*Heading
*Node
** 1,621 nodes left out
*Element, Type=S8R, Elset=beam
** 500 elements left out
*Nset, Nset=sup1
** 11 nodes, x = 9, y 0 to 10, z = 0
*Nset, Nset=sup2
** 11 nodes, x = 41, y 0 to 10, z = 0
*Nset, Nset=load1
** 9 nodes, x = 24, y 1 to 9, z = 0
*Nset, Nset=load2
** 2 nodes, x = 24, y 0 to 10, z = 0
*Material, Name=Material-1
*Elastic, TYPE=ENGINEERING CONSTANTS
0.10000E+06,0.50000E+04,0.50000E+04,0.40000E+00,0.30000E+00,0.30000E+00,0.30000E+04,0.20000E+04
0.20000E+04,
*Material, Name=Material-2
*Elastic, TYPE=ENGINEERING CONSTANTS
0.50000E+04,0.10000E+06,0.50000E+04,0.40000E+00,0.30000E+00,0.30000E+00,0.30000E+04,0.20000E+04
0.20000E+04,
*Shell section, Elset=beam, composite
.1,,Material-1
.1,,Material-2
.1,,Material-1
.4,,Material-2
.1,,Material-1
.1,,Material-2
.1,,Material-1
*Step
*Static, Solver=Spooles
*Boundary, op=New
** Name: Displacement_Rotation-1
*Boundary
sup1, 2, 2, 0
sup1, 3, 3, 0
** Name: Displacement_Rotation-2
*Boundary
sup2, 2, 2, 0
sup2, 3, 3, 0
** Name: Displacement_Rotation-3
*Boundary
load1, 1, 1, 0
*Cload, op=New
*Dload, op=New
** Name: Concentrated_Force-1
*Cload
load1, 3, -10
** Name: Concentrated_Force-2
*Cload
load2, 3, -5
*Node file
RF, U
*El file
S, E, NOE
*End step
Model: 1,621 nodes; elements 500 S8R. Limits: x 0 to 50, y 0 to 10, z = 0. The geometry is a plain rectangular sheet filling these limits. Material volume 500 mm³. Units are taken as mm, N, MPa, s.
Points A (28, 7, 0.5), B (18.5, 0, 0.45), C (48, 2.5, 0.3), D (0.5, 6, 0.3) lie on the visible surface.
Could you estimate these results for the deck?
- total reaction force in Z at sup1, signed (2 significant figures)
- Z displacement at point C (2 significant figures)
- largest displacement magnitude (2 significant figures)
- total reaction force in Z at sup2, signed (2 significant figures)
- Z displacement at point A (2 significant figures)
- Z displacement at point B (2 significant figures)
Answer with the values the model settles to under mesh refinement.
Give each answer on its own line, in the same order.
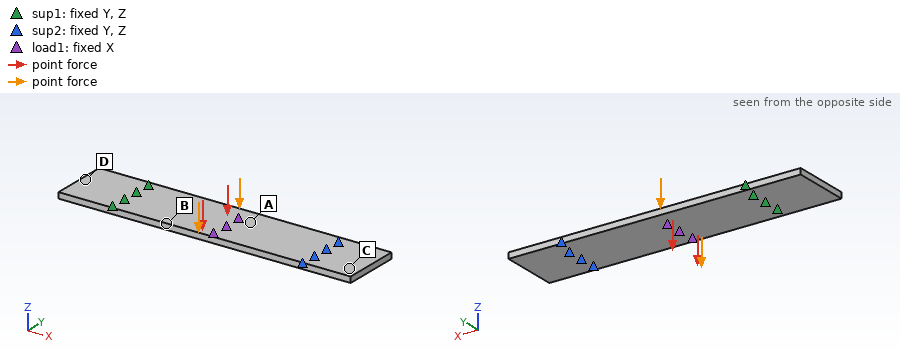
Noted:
53 N
0.79 mm
1.3 mm
47 N
-1.2 mm
-1.1 mm
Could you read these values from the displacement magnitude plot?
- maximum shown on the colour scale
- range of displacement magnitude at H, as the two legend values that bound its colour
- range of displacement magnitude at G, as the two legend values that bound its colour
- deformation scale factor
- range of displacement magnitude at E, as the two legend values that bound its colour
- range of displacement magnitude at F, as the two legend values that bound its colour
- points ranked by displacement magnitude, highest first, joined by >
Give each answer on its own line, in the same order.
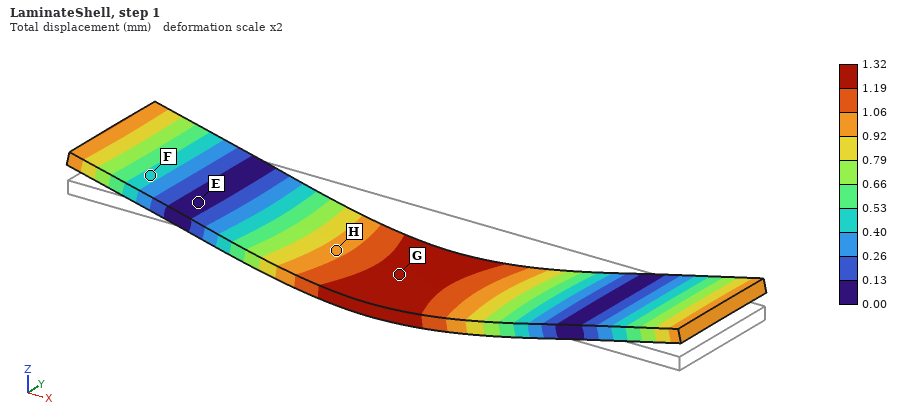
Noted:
1.32 mm
0.92 to 1.06 mm
1.19 to 1.32 mm
2
0.00 to 0.13 mm
0.40 to 0.53 mm
G > H > F > E
